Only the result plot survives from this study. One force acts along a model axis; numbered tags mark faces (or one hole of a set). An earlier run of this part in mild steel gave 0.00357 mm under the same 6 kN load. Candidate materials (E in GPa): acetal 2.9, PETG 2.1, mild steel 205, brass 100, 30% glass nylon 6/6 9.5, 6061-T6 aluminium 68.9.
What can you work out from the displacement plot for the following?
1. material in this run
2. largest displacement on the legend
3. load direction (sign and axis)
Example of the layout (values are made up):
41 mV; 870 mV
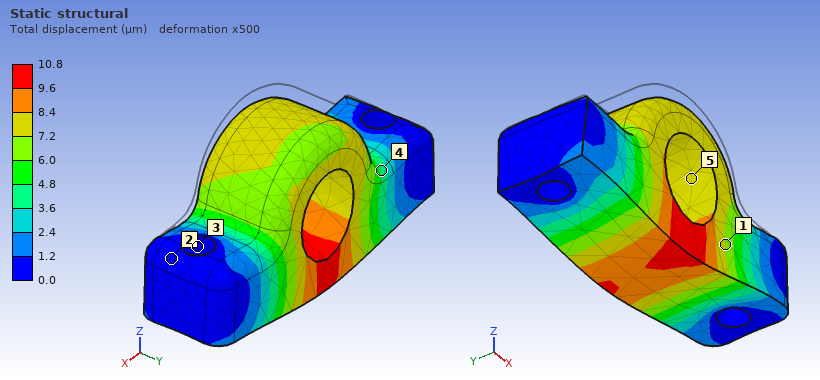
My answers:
6061-T6 aluminium; 10.8 µm; -Z
